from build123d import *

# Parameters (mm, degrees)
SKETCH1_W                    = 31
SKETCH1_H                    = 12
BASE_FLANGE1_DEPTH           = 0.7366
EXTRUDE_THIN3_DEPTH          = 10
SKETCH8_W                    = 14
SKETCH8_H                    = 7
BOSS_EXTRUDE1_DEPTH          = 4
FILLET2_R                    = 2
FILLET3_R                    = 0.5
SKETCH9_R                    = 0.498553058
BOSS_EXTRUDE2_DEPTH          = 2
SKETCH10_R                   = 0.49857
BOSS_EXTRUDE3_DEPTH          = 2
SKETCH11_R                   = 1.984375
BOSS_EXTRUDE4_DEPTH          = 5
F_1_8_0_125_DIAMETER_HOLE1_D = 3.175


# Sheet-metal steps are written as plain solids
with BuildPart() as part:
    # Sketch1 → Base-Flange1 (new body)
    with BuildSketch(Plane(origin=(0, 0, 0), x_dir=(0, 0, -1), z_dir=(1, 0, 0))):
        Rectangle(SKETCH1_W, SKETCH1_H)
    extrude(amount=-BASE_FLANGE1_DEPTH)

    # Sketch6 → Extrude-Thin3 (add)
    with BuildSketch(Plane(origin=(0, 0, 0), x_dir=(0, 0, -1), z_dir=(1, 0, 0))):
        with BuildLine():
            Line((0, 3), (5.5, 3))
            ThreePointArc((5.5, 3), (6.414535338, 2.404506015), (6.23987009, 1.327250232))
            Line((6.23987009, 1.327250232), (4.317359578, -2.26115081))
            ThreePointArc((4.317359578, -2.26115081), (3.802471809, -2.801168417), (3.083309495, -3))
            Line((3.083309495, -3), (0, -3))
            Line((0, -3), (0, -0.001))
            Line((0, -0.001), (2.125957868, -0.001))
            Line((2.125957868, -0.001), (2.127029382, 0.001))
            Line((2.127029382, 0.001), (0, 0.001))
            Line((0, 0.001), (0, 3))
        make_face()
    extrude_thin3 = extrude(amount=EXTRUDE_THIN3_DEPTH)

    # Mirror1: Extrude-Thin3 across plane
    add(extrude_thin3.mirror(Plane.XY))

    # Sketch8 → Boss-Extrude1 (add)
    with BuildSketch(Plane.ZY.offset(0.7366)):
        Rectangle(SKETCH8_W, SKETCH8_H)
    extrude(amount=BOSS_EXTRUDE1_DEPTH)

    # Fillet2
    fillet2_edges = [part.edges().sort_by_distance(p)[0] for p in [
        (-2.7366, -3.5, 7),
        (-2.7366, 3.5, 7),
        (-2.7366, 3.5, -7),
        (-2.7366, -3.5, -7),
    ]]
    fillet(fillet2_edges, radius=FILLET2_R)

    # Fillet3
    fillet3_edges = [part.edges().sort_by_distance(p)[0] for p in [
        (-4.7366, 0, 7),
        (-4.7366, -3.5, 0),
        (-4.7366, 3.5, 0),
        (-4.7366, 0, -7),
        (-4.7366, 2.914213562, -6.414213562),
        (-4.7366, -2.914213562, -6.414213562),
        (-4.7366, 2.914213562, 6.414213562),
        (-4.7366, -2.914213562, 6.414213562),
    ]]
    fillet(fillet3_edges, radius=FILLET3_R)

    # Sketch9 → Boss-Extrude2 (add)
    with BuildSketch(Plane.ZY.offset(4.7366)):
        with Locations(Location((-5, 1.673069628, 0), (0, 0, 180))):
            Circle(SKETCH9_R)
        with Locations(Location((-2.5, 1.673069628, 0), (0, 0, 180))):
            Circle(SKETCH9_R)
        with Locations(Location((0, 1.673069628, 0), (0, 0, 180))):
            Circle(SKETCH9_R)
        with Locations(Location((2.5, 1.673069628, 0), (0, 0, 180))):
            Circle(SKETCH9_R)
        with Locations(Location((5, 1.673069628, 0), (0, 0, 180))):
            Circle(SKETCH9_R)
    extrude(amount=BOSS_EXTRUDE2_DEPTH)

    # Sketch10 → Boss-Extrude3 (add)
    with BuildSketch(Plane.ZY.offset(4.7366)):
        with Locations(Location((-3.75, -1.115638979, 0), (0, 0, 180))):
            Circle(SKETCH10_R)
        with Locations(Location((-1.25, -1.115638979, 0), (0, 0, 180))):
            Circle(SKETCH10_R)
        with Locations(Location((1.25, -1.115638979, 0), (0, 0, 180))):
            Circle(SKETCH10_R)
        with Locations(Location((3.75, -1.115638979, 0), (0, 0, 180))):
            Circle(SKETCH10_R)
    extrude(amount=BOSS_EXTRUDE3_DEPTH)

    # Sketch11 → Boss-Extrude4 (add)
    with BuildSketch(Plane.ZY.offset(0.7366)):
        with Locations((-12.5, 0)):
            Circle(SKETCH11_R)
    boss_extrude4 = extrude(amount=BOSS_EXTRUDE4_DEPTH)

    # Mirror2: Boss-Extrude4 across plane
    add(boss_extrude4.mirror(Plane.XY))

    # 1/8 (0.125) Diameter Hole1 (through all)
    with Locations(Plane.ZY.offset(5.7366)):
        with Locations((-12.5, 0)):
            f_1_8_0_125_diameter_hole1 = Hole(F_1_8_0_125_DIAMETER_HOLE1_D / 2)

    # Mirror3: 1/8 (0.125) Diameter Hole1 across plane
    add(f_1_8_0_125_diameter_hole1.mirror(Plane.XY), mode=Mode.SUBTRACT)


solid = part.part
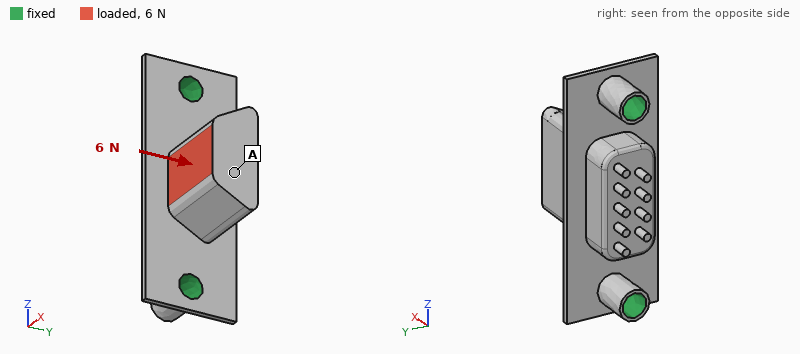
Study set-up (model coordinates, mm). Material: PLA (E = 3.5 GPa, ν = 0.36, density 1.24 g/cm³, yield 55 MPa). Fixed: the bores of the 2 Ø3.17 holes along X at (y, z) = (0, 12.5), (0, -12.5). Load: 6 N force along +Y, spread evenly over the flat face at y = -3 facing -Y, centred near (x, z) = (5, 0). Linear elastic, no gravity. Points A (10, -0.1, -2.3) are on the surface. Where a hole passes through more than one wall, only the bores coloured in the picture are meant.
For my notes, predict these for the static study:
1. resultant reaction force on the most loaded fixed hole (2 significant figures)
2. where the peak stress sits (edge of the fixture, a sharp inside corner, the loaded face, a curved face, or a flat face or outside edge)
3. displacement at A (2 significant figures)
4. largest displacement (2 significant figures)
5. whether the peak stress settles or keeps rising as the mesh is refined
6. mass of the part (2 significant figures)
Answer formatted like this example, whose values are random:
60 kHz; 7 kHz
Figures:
3.0 N; edge of the fixture; 0.23 mm; 0.24 mm; keeps rising; 1.7 g
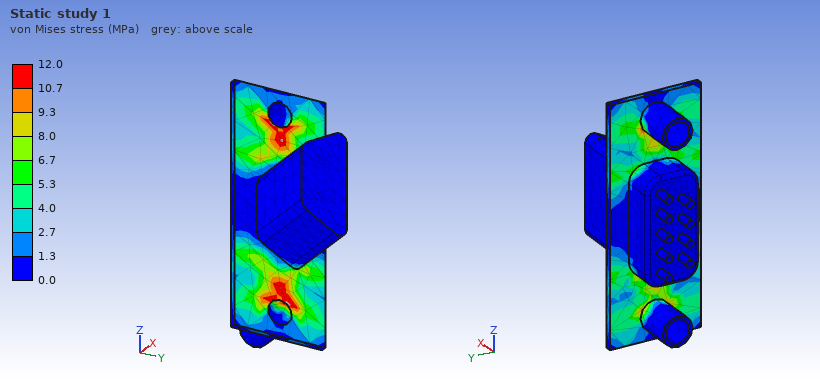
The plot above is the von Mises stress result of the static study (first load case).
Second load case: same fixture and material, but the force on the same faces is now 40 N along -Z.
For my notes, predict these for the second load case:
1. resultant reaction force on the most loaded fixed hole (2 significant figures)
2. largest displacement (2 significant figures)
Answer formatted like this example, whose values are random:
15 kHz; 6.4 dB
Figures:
24 N; 0.15 mm
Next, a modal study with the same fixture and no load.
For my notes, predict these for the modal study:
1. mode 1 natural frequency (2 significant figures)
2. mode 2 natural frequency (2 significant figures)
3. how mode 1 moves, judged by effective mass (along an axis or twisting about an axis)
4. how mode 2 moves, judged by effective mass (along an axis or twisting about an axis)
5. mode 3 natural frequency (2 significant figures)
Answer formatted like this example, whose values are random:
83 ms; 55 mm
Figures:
960 Hz; 2000 Hz; along Y; along X; 2900 Hz
